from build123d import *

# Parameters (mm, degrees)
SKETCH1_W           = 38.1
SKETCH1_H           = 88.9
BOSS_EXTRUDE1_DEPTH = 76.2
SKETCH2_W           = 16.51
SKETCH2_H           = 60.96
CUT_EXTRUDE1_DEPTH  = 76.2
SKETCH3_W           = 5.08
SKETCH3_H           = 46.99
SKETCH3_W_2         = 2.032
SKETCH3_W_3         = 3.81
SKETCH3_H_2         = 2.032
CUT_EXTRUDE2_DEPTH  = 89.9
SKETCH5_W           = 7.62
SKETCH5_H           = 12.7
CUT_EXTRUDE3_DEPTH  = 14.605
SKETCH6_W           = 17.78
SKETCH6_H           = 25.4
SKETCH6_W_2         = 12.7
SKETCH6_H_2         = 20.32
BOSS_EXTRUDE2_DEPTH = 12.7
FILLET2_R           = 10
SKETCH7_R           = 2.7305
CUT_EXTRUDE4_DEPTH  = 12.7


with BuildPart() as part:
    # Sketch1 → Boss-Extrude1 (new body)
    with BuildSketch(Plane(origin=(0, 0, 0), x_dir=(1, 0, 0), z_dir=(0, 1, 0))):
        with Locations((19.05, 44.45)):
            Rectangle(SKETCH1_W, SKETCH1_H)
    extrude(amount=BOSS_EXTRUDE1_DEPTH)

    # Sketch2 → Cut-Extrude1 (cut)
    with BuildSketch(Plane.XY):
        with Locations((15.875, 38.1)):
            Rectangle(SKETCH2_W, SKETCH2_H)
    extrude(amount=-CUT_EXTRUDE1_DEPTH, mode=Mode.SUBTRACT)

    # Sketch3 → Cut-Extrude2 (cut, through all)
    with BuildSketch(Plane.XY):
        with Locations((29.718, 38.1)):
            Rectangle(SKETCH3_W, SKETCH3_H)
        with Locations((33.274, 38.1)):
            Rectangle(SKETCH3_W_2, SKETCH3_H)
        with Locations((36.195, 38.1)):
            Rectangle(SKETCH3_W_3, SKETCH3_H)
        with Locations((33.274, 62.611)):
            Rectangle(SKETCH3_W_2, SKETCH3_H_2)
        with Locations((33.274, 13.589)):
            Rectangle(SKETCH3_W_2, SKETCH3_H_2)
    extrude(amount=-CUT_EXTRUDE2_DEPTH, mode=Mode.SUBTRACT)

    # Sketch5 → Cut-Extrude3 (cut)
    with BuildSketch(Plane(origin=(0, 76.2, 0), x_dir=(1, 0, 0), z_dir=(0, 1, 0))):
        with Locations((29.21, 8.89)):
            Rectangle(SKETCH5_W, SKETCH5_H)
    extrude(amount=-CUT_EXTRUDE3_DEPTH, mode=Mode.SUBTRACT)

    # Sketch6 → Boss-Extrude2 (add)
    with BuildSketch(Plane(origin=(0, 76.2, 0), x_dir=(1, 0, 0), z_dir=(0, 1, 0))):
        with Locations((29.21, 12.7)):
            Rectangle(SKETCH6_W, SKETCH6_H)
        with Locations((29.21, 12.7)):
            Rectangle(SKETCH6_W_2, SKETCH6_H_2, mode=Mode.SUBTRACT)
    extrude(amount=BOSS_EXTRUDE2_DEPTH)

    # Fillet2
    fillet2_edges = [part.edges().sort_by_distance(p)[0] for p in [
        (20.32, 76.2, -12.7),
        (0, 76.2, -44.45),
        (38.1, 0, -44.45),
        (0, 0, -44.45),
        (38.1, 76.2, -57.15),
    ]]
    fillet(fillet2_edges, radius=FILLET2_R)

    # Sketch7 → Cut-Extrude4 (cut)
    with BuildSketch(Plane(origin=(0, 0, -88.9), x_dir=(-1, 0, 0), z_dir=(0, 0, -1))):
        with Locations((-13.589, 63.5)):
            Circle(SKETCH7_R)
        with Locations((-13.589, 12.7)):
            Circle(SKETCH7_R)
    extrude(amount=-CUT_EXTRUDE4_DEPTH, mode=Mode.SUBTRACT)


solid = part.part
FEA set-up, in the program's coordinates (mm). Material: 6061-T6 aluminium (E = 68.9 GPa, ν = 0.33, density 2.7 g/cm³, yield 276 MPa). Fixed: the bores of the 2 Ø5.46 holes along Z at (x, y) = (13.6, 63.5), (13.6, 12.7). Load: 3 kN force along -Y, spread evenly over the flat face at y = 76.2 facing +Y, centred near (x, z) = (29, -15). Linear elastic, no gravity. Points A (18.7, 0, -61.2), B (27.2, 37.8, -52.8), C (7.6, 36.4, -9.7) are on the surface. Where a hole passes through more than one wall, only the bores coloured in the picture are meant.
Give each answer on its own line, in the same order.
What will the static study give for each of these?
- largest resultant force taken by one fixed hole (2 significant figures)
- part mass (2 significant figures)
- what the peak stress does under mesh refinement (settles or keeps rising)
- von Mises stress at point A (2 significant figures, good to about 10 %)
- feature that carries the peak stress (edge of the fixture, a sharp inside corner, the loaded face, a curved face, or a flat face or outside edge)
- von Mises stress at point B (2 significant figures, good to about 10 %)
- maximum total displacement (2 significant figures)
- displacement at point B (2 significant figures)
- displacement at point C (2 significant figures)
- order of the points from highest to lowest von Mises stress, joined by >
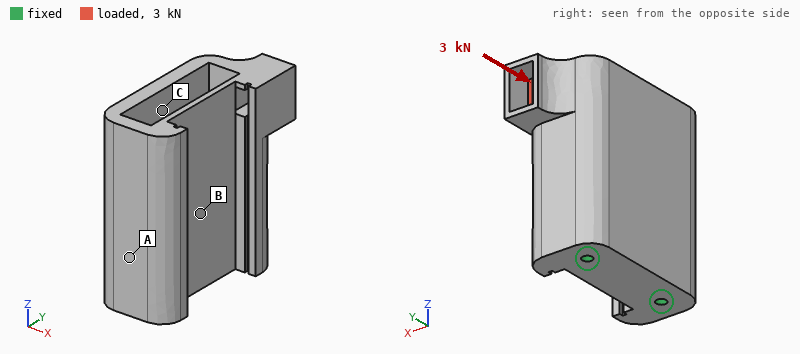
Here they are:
3.9 kN
350 g
keeps rising
10 MPa
a sharp inside corner
18 MPa
95 µm
17 µm
19 µm
B > A > C
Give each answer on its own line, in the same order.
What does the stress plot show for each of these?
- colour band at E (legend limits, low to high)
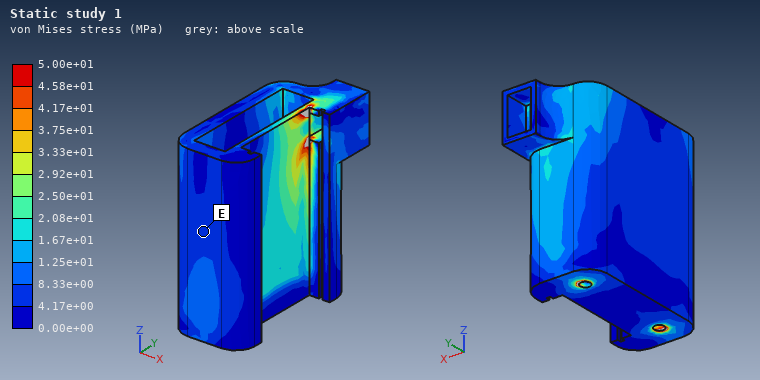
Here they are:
4.17e+00 to 8.33e+00 MPa
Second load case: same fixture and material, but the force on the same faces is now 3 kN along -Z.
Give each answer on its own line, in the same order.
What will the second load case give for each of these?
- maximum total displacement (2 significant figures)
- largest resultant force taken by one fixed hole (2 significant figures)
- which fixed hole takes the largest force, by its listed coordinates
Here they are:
85 µm
3.5 kN
(13.6, 63.5)
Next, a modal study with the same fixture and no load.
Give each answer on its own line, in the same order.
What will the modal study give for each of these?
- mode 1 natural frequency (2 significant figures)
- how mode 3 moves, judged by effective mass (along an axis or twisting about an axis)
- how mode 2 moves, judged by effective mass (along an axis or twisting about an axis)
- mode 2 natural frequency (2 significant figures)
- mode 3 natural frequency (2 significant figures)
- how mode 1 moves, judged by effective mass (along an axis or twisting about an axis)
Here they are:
1700 Hz
along Y
twisting about Z
3300 Hz
4000 Hz
along X
